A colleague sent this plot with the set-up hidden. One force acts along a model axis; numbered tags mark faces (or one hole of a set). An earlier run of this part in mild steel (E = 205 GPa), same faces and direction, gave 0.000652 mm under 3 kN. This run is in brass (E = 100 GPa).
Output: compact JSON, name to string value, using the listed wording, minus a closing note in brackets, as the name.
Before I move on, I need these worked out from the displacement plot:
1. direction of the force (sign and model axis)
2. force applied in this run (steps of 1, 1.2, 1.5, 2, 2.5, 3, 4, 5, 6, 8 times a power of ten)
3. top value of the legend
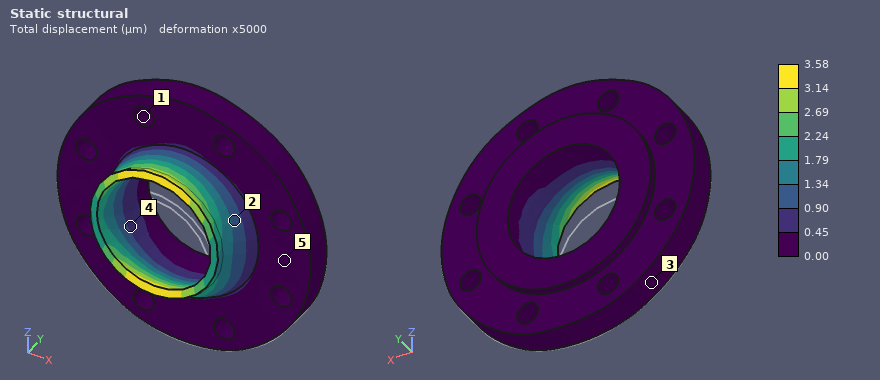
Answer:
{"direction of the force": "+Z", "force applied in this run": "8 kN", "top value of the legend": "3.58 µm"}
